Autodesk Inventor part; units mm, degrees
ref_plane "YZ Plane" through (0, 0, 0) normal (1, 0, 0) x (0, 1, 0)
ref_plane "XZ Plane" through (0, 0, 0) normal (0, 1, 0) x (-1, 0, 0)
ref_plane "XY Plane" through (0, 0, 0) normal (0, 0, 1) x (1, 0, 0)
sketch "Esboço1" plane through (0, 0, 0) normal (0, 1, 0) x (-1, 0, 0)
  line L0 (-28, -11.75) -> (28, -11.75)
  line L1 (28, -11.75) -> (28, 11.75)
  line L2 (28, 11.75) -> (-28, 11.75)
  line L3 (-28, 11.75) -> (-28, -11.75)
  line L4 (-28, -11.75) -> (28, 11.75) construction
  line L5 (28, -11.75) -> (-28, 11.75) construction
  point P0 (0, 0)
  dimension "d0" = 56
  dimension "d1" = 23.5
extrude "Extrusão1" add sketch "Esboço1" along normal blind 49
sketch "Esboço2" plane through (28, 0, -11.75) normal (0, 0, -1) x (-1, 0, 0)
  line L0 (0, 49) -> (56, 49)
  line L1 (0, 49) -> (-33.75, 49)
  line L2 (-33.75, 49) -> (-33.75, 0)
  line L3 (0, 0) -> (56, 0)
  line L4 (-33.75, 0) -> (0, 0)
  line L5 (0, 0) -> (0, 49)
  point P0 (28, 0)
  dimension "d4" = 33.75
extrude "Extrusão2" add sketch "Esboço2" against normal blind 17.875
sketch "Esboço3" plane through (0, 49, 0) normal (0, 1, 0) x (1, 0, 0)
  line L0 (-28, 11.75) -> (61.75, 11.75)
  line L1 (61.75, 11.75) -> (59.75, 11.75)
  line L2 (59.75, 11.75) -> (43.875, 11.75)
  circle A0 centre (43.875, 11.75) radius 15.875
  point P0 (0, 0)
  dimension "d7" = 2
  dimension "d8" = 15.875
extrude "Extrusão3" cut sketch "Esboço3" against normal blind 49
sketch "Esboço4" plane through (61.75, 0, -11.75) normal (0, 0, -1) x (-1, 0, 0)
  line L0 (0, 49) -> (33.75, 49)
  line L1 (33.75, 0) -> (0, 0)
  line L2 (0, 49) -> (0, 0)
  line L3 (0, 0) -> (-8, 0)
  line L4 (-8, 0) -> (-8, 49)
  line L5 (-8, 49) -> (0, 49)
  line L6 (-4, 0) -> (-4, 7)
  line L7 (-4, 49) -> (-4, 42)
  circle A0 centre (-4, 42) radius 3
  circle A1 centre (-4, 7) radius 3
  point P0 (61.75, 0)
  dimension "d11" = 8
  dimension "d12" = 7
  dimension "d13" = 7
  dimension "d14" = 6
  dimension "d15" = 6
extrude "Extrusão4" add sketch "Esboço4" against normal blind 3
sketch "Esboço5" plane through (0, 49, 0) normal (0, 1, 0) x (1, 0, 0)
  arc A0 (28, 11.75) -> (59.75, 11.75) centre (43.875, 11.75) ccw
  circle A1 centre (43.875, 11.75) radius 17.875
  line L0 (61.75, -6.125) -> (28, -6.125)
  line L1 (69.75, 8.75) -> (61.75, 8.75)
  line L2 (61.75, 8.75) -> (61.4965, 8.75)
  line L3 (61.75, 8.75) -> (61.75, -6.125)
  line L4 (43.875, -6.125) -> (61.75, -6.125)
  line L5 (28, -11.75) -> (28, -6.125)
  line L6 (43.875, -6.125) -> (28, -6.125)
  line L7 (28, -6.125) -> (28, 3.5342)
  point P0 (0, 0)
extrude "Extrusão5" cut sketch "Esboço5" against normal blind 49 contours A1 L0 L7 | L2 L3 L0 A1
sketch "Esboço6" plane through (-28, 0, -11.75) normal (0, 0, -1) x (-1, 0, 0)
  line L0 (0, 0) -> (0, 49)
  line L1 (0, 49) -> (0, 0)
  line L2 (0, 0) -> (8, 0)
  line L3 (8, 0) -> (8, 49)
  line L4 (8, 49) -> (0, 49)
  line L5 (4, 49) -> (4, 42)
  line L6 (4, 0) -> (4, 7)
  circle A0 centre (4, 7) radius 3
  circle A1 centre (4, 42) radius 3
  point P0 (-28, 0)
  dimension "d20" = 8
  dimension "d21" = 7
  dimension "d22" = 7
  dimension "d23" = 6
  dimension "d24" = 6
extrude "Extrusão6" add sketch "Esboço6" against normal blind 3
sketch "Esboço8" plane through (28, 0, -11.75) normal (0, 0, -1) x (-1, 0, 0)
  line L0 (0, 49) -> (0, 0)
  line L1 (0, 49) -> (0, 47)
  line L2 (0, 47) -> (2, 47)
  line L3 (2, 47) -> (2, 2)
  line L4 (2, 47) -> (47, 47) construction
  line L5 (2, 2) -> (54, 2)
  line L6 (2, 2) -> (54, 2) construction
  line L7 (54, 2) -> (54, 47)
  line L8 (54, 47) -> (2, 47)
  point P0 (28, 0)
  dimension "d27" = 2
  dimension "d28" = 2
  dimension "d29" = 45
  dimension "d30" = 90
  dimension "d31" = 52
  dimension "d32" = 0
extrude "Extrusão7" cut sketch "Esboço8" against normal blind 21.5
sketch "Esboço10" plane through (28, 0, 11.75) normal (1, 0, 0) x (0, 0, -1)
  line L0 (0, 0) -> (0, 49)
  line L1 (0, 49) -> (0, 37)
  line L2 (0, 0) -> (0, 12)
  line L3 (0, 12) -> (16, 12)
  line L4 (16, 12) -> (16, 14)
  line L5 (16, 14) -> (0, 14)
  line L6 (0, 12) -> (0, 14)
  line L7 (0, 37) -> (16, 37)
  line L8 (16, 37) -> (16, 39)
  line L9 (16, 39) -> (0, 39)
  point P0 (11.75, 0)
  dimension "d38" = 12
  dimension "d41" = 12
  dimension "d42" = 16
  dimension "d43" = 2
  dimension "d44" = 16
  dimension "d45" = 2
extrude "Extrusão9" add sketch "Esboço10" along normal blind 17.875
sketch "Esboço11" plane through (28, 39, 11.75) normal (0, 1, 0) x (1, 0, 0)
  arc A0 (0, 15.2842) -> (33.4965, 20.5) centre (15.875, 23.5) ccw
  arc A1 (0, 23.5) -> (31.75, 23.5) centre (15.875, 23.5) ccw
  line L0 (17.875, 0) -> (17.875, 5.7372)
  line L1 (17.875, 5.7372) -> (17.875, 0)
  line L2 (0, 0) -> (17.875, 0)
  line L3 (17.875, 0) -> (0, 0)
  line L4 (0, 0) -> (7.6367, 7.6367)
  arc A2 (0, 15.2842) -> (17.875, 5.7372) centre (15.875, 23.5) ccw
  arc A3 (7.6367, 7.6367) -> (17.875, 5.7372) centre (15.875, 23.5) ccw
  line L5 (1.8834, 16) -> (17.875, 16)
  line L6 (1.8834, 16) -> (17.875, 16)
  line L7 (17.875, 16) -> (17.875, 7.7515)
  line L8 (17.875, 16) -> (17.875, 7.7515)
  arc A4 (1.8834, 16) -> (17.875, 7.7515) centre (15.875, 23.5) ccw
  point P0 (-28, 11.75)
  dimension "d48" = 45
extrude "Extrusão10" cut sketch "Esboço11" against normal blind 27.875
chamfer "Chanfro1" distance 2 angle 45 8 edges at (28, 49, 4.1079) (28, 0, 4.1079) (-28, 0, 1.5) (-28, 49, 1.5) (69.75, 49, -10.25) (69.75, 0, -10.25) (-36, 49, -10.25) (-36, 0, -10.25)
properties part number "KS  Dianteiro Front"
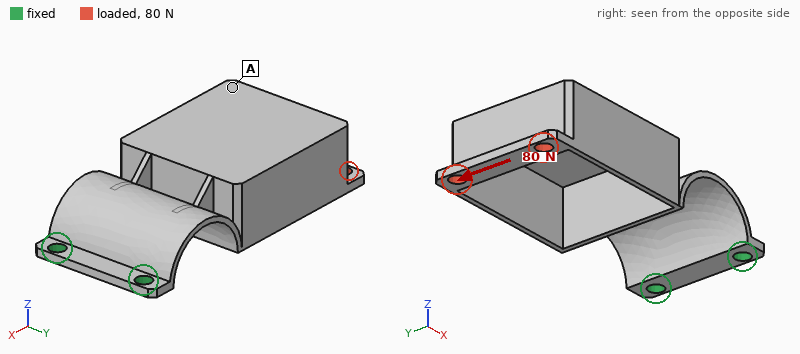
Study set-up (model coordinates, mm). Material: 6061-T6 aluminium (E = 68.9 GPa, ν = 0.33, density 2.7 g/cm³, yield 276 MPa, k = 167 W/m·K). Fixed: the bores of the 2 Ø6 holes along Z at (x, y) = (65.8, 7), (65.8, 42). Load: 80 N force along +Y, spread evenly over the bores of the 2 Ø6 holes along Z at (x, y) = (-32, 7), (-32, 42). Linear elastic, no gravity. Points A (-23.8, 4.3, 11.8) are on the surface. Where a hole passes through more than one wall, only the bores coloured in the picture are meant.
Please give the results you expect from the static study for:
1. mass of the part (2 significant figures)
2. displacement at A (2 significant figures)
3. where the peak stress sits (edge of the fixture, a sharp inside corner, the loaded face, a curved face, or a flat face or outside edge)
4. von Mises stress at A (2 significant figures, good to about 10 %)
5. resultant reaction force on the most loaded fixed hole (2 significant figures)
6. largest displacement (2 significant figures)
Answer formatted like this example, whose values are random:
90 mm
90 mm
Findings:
56 g
0.72 mm
a curved face
8.7 MPa
210 N
1.2 mm
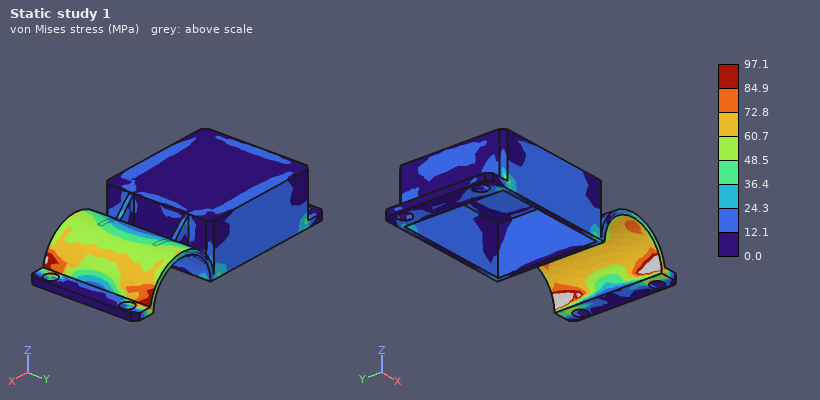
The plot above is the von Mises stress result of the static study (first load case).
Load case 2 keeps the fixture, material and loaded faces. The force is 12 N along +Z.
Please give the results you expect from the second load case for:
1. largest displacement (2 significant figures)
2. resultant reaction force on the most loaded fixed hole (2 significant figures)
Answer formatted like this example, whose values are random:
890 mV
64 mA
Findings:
1.3 mm
22 N
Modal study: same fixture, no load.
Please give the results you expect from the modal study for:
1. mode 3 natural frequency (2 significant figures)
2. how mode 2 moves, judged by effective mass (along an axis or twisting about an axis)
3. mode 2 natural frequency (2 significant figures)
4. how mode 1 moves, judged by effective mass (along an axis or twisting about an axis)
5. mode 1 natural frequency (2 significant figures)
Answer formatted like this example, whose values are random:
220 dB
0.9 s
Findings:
830 Hz
along Y
340 Hz
along Z
110 Hz
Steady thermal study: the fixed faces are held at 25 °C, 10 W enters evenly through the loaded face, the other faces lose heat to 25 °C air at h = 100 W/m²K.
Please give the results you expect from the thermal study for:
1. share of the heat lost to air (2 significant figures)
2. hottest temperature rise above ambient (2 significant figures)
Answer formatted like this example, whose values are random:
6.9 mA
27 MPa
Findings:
94 %
19 K
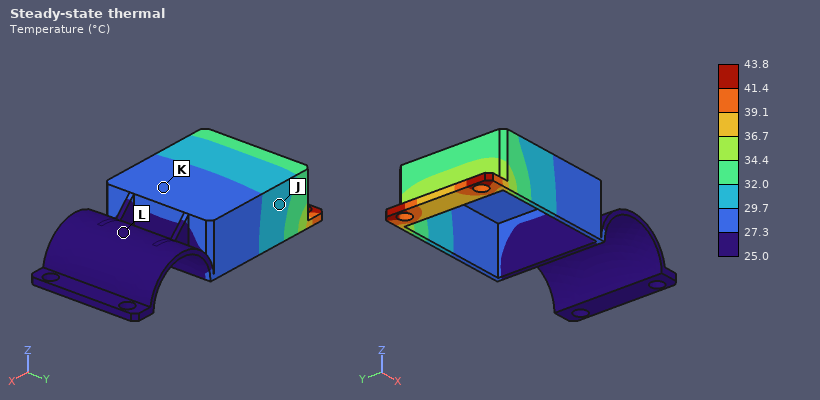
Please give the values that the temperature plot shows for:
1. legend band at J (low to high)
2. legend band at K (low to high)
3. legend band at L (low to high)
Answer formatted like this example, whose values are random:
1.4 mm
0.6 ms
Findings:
29.7 to 32.0 °C
27.3 to 29.7 °C
25.0 to 27.3 °C
